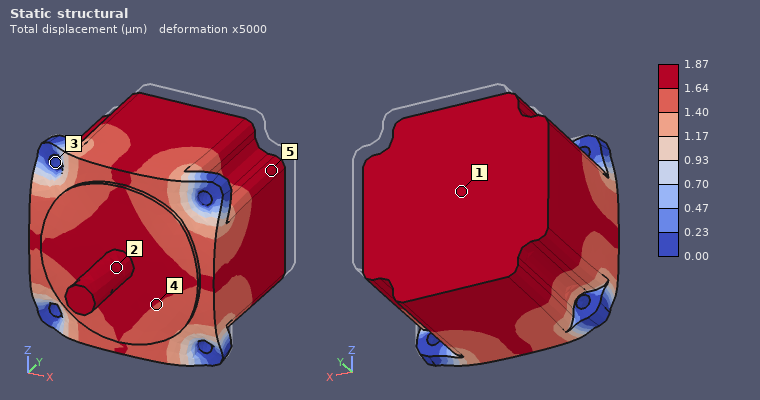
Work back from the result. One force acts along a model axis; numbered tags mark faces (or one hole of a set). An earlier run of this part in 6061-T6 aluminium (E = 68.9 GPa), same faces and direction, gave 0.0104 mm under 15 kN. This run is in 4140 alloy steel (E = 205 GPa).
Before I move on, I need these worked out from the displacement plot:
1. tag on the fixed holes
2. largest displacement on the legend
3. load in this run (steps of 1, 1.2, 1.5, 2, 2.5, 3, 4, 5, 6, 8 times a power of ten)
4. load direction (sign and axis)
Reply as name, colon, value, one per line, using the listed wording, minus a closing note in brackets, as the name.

tag on the fixed holes: 3
largest displacement on the legend: 1.87 µm
load in this run: 8 kN
load direction: -Y
